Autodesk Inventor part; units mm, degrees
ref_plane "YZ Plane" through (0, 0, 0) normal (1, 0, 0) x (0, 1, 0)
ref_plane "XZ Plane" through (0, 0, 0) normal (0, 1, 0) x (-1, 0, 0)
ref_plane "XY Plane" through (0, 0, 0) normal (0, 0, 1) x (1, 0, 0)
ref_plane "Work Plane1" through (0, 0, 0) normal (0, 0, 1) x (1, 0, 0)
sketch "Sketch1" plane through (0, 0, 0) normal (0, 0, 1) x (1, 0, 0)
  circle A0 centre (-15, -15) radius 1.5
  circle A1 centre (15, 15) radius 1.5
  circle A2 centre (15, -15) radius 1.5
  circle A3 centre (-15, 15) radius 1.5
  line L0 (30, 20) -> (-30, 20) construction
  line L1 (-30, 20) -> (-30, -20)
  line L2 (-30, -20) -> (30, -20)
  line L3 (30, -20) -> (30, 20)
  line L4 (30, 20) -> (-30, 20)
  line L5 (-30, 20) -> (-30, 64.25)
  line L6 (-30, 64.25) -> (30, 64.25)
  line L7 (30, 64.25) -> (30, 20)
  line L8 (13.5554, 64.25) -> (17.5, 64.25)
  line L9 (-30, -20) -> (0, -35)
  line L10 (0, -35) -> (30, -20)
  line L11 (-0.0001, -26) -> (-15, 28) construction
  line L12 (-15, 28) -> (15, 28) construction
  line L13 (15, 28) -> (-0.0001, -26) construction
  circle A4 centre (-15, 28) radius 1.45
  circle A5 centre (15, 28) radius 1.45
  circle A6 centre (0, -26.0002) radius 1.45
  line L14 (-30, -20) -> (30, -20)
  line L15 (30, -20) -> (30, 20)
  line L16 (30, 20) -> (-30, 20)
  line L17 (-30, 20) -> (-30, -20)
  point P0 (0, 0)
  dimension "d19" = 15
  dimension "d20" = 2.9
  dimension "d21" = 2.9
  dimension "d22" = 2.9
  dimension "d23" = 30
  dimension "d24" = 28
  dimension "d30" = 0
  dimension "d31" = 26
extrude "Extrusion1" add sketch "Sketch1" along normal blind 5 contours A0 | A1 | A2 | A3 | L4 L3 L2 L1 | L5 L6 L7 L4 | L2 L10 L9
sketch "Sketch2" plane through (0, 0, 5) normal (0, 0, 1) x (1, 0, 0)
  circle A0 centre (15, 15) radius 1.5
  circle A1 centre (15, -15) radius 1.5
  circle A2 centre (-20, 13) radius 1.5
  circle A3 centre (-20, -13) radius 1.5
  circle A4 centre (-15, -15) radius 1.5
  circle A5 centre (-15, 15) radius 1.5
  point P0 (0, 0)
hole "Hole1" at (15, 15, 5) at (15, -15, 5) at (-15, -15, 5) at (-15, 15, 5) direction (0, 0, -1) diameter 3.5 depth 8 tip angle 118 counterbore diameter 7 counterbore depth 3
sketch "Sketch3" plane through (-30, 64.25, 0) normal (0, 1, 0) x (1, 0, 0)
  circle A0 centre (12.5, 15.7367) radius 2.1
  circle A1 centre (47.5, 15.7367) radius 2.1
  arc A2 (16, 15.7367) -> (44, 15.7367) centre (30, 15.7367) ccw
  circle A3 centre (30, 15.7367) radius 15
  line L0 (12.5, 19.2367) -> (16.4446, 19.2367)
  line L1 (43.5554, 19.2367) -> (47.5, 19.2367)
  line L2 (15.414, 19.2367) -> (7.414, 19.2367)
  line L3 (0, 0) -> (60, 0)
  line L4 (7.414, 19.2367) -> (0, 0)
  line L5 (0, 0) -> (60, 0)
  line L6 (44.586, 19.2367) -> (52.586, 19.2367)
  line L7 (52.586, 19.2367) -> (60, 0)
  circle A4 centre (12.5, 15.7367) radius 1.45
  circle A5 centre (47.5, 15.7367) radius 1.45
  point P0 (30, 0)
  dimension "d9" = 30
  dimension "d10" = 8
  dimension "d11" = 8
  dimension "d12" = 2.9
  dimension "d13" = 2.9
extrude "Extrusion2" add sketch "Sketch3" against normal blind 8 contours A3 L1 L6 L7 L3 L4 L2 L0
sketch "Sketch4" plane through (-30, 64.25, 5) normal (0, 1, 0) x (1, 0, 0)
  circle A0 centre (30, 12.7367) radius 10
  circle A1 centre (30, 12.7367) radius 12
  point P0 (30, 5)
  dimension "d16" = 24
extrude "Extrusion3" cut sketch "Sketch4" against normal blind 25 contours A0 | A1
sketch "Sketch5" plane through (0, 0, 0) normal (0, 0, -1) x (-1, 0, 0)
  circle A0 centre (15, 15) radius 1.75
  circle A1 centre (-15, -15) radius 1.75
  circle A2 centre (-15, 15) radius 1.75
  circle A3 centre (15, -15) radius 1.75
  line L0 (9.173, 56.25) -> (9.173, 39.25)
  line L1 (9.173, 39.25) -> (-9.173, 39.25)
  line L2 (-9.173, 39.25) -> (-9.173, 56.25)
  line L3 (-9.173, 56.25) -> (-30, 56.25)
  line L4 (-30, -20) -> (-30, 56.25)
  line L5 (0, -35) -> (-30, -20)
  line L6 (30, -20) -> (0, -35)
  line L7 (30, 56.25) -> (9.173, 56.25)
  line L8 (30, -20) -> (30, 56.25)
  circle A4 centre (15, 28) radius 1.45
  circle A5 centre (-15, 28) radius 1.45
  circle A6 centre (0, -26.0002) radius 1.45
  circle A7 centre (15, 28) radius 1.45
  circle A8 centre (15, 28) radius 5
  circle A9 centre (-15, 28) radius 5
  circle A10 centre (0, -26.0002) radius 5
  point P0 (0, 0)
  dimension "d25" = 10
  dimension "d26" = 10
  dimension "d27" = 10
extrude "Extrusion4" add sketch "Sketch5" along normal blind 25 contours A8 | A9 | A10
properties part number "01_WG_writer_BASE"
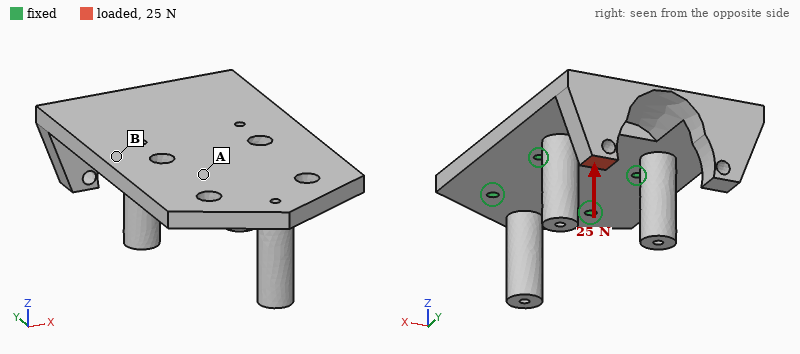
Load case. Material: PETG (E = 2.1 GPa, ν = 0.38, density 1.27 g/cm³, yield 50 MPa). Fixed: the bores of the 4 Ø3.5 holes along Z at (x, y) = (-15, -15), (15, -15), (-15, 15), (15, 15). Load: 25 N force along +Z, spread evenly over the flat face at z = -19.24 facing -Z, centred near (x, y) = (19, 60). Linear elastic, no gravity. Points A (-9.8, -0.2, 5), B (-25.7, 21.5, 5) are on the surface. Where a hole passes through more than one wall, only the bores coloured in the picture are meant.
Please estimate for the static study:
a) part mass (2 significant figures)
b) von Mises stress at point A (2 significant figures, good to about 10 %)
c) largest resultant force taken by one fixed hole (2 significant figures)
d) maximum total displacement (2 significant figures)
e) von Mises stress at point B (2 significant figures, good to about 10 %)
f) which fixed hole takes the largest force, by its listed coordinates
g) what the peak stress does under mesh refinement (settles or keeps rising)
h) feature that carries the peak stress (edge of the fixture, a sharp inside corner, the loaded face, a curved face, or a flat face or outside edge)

44 g
1.2 MPa
72 N
1.4 mm
2.9 MPa
(15, 15)
keeps rising
edge of the fixture
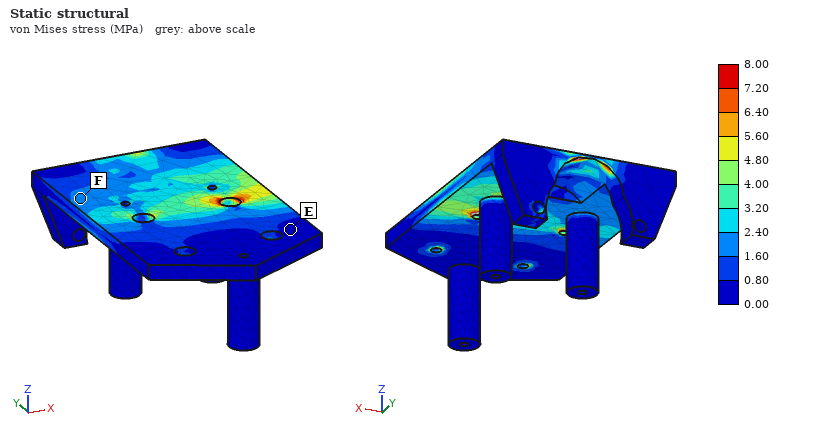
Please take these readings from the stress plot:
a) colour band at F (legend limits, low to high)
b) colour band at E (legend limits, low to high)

1.60 to 2.40 MPa
0.00 to 0.80 MPa
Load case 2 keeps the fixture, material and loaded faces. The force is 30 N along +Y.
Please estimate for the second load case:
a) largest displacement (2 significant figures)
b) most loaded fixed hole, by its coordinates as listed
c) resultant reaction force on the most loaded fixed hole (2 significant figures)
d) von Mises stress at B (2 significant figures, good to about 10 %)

1.3 mm
(15, 15)
51 N
2.1 MPa
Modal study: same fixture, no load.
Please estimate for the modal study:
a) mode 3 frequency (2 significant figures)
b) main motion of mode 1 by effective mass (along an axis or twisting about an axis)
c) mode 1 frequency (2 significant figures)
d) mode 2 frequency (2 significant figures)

910 Hz
along Z
270 Hz
460 Hz
